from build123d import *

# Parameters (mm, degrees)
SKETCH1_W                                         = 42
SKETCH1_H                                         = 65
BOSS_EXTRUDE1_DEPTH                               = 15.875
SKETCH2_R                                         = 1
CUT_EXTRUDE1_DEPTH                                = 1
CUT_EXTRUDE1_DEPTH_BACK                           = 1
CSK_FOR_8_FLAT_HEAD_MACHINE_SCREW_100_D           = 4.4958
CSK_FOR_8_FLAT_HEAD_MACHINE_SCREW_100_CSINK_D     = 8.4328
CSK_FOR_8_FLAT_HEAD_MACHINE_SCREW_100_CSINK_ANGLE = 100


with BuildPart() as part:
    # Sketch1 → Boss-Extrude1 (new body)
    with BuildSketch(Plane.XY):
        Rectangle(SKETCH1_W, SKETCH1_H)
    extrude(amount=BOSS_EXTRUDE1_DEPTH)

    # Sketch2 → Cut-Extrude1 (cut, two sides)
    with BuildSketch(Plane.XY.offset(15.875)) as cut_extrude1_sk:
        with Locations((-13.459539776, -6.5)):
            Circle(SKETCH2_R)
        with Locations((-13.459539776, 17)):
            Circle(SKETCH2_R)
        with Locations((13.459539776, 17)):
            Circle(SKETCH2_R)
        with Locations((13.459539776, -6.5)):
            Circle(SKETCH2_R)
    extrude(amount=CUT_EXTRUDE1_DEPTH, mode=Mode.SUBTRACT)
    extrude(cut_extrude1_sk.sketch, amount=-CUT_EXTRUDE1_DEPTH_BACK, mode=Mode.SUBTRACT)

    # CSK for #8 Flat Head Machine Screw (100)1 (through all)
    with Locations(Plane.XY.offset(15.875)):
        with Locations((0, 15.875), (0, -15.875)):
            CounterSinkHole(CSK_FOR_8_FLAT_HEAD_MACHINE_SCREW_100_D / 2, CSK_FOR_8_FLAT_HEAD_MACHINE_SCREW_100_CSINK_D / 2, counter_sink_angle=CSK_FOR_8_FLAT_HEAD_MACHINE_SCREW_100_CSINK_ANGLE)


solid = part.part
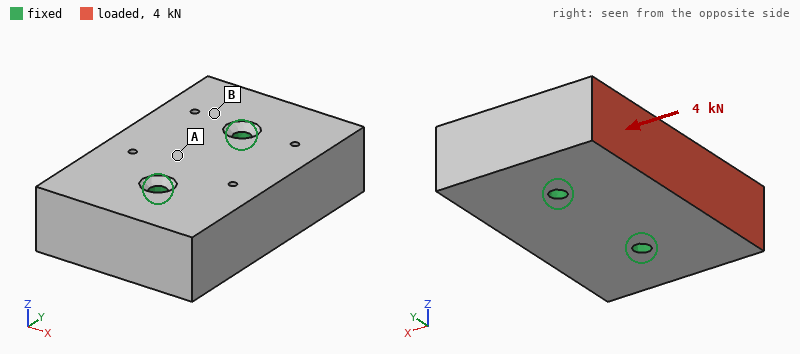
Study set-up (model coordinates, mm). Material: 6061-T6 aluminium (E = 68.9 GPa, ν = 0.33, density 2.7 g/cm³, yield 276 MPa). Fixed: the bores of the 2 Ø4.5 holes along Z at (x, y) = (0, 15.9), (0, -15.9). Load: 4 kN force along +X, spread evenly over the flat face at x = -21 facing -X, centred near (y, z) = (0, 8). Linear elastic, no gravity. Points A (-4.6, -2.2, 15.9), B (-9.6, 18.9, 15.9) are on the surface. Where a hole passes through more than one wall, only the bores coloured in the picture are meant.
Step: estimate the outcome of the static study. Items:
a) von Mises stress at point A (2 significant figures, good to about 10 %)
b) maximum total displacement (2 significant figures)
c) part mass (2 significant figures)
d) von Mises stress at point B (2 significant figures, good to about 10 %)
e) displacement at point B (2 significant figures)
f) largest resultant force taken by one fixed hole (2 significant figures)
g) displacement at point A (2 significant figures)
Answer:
1.9 MPa
2.7 µm
120 g
5.1 MPa
1.2 µm
2.0 kN
1.0 µm
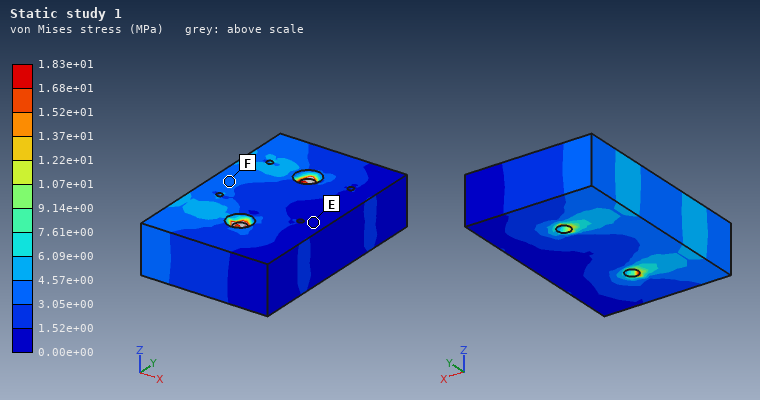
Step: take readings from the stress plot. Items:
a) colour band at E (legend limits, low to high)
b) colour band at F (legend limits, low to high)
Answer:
0.00e+00 to 1.52e+00 MPa
3.05e+00 to 4.57e+00 MPa
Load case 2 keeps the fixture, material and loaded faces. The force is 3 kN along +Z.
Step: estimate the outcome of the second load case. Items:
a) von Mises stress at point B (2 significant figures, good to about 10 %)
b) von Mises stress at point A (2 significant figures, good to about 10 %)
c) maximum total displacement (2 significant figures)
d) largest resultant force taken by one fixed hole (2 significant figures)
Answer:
13 MPa
9.9 MPa
17 µm
1.5 kN
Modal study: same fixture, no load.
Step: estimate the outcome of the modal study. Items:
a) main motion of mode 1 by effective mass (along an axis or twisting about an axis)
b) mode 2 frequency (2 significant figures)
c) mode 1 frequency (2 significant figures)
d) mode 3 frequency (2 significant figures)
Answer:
twisting about Y
18 kHz
13 kHz
18 kHz
